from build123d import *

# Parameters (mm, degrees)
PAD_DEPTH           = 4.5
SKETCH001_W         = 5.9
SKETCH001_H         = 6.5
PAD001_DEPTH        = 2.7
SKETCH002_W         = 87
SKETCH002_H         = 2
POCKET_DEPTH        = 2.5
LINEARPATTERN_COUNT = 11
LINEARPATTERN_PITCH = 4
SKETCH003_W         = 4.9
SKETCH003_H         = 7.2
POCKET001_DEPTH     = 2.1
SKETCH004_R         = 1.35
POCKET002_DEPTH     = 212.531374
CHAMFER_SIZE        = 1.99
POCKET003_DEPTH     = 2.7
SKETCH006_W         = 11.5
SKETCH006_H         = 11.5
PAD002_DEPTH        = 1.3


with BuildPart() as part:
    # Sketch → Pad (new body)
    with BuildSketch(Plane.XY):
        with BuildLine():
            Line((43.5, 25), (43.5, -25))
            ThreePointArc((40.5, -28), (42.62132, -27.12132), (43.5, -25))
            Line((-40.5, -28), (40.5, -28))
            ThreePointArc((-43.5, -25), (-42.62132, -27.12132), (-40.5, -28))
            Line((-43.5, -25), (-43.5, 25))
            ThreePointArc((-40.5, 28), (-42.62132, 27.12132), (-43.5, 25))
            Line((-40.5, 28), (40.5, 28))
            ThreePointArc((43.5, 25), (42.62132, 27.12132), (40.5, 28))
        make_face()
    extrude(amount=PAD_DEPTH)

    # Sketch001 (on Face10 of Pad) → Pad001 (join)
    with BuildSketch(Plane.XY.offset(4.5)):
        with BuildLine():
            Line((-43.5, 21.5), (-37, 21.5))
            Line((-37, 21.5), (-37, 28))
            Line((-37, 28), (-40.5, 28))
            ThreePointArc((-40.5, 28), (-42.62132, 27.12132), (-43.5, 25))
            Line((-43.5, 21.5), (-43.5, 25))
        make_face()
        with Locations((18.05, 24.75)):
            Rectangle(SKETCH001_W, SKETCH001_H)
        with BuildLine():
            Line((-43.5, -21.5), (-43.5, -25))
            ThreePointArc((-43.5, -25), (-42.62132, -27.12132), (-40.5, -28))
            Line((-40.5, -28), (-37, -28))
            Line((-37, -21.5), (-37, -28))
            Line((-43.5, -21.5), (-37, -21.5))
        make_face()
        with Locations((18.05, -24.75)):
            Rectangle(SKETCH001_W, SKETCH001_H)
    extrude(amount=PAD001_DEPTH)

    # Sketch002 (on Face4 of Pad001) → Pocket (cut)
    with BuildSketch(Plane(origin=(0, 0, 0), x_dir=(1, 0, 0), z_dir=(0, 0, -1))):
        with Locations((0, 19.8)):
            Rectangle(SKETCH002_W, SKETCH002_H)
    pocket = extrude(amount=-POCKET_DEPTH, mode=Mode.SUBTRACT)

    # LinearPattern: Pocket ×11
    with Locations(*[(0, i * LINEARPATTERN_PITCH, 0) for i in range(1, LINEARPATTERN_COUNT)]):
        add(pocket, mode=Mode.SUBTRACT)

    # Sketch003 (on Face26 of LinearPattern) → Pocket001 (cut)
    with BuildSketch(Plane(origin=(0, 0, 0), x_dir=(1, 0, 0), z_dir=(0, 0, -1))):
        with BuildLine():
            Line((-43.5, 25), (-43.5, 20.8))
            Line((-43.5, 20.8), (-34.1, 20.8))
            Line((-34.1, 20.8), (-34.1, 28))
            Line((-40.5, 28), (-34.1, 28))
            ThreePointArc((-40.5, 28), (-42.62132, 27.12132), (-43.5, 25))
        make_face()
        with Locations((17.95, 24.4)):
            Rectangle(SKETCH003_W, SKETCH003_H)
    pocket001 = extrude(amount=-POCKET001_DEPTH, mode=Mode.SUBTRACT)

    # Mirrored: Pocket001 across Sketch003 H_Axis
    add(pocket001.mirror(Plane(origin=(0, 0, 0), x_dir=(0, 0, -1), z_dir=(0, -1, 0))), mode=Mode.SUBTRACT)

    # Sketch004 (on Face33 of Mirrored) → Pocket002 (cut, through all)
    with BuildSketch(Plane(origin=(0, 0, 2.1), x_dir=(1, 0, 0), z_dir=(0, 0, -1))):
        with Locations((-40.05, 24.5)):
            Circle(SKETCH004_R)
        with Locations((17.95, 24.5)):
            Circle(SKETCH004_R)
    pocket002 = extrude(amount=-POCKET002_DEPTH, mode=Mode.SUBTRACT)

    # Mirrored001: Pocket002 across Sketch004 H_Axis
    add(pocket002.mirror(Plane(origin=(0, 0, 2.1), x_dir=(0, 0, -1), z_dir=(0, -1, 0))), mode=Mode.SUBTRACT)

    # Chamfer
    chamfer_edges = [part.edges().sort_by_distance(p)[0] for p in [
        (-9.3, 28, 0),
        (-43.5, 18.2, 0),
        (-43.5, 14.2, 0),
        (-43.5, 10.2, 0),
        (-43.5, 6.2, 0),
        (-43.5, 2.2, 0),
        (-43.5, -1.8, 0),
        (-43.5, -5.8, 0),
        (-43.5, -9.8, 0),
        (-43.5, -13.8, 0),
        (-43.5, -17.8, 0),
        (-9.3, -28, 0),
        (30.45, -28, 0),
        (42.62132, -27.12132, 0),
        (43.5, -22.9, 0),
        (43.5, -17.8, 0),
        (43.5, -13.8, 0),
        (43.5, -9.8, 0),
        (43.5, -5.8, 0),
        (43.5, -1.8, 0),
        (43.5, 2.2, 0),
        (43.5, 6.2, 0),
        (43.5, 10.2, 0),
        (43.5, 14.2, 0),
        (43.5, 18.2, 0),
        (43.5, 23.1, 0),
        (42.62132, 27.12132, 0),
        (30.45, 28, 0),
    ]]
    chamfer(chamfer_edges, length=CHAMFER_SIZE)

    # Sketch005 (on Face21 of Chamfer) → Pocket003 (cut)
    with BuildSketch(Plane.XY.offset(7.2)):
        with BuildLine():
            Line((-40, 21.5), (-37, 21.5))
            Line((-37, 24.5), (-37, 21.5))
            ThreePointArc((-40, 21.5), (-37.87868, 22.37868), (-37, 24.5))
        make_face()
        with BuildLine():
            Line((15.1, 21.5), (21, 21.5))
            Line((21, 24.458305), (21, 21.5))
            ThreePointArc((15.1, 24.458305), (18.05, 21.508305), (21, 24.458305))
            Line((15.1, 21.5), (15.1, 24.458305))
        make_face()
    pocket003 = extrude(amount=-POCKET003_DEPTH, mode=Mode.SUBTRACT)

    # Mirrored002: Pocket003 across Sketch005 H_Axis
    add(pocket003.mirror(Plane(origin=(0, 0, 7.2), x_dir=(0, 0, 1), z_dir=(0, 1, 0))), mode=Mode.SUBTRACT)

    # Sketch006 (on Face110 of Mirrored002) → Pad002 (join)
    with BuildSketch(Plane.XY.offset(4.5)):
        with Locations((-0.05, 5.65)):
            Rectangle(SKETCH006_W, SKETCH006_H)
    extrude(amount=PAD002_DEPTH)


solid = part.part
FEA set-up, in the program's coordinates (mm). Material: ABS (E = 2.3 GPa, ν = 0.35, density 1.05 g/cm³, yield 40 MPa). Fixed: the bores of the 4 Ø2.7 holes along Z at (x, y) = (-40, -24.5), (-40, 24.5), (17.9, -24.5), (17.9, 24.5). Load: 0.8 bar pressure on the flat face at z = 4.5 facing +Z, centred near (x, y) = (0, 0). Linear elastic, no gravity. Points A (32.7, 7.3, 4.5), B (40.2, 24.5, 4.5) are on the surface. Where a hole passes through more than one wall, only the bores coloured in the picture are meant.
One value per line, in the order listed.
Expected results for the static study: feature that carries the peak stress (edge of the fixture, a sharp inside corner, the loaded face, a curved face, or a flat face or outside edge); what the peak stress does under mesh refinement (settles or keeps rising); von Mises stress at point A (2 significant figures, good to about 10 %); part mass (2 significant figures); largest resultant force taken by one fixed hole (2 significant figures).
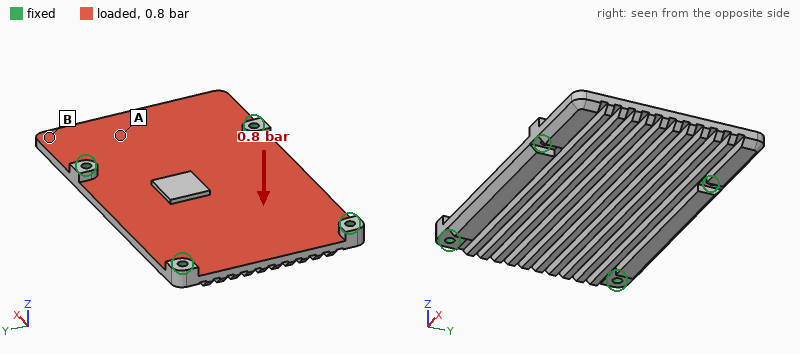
edge of the fixture
keeps rising
7.6 MPa
18 g
130 N
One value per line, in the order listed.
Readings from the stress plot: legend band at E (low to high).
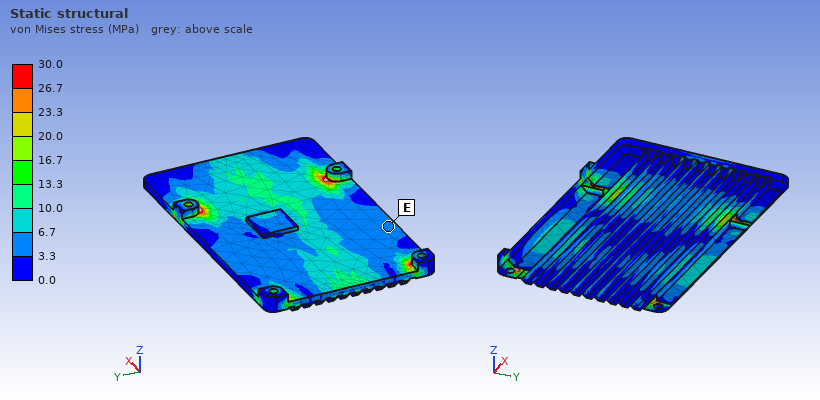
3.3 to 6.7 MPa
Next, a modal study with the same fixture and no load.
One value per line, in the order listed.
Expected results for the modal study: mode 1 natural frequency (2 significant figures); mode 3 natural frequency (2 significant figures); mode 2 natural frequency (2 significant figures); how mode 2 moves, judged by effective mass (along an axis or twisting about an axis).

860 Hz
1400 Hz
910 Hz
along Z
